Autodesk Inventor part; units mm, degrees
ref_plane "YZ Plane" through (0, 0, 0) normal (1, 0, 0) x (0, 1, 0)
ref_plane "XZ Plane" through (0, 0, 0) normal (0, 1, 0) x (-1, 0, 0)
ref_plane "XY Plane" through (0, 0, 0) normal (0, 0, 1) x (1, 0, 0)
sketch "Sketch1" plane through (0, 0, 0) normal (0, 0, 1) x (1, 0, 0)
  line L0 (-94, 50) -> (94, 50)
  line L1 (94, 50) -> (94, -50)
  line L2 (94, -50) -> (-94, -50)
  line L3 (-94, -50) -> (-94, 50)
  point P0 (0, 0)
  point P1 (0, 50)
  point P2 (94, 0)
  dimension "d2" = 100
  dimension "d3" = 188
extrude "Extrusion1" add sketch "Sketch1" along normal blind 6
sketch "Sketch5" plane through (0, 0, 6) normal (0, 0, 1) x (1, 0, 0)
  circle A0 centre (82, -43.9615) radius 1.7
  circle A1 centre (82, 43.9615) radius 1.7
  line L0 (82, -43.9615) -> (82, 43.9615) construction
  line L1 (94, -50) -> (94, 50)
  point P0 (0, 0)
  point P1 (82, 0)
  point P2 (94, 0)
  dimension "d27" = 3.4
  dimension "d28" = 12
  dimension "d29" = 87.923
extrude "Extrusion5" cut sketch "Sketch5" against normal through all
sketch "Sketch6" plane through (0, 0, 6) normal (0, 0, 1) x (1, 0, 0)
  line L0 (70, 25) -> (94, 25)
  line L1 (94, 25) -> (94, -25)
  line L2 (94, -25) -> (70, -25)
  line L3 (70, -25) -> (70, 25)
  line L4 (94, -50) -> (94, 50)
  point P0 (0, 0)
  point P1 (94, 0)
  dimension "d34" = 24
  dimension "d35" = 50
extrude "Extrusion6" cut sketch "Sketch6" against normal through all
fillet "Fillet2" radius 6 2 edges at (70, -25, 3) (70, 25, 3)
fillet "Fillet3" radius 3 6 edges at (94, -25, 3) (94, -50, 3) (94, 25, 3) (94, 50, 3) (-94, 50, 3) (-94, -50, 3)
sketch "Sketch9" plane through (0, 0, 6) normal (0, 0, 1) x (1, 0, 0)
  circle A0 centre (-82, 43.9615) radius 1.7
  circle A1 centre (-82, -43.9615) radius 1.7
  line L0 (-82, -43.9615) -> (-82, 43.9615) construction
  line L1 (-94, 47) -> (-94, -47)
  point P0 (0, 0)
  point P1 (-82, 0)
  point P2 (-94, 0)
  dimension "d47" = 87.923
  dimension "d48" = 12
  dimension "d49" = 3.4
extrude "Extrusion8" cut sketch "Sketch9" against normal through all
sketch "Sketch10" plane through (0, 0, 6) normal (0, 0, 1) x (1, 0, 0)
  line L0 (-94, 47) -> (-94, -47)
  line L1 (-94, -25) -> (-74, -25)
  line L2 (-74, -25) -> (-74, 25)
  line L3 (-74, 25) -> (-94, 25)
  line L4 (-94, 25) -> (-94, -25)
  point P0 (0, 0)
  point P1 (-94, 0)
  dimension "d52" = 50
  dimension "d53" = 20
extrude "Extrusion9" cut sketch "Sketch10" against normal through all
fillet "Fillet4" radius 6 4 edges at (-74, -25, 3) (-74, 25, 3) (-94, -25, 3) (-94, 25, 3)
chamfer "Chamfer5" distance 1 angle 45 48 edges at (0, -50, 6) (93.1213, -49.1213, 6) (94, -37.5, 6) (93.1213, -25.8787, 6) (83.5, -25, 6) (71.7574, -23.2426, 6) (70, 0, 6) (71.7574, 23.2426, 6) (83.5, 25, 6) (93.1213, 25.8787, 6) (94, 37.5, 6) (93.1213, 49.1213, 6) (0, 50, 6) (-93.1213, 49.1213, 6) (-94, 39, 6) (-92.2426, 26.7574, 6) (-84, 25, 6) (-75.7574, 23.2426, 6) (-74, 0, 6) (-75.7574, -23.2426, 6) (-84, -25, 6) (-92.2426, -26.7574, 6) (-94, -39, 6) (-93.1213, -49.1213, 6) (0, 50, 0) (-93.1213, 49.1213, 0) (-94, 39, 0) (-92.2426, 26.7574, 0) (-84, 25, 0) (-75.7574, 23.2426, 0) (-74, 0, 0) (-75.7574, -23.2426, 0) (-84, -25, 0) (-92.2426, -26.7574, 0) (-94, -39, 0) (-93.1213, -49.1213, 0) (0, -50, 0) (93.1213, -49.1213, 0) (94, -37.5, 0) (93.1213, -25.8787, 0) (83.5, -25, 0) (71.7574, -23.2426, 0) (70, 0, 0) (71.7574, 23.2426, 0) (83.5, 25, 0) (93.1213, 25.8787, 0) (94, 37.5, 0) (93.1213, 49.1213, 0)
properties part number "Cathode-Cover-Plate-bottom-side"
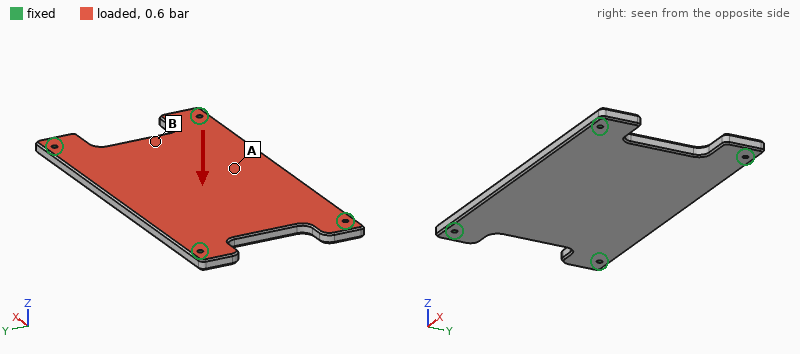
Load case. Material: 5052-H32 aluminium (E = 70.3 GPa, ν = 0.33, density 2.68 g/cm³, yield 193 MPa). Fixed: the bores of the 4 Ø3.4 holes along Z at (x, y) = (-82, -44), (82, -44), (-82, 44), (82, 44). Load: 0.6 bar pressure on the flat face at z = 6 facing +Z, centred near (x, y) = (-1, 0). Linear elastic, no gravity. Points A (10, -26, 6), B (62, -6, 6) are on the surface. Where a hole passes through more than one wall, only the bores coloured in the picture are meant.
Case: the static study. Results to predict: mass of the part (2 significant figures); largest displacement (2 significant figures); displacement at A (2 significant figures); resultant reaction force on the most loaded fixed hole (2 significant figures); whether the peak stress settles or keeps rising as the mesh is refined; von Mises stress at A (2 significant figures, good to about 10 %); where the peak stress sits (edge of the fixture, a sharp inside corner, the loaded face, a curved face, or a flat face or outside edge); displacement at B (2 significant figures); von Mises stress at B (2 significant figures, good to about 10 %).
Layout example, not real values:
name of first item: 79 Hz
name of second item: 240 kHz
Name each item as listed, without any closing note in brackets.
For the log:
mass of the part: 260 g
largest displacement: 0.15 mm
displacement at A: 0.14 mm
resultant reaction force on the most loaded fixed hole: 240 N
whether the peak stress settles or keeps rising as the mesh is refined: keeps rising
von Mises stress at A: 13 MPa
where the peak stress sits: edge of the fixture
displacement at B: 0.053 mm
von Mises stress at B: 5.6 MPa
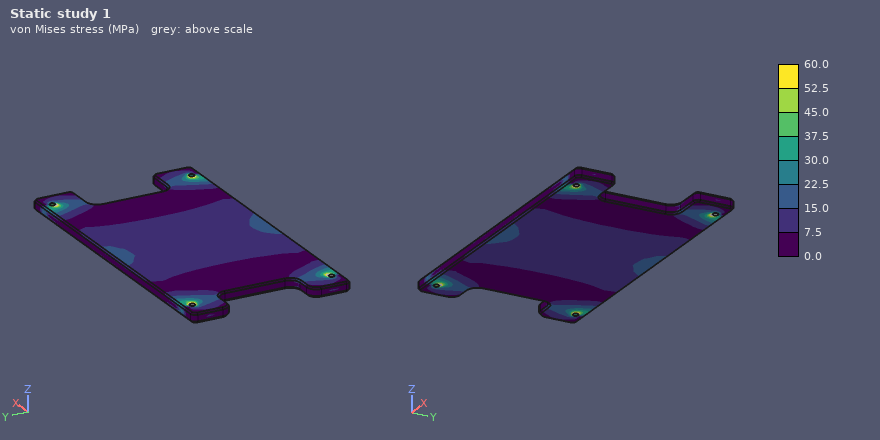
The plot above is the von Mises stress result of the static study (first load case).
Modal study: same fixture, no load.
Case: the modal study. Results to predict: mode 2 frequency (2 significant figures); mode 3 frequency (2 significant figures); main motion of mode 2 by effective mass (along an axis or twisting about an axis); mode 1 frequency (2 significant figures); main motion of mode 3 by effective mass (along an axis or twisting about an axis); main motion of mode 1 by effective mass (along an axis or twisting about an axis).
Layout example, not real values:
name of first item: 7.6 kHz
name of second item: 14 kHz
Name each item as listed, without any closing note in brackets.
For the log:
mode 2 frequency: 1600 Hz
mode 3 frequency: 2500 Hz
main motion of mode 2 by effective mass: twisting about X
mode 1 frequency: 900 Hz
main motion of mode 3 by effective mass: twisting about Y
main motion of mode 1 by effective mass: along Z
